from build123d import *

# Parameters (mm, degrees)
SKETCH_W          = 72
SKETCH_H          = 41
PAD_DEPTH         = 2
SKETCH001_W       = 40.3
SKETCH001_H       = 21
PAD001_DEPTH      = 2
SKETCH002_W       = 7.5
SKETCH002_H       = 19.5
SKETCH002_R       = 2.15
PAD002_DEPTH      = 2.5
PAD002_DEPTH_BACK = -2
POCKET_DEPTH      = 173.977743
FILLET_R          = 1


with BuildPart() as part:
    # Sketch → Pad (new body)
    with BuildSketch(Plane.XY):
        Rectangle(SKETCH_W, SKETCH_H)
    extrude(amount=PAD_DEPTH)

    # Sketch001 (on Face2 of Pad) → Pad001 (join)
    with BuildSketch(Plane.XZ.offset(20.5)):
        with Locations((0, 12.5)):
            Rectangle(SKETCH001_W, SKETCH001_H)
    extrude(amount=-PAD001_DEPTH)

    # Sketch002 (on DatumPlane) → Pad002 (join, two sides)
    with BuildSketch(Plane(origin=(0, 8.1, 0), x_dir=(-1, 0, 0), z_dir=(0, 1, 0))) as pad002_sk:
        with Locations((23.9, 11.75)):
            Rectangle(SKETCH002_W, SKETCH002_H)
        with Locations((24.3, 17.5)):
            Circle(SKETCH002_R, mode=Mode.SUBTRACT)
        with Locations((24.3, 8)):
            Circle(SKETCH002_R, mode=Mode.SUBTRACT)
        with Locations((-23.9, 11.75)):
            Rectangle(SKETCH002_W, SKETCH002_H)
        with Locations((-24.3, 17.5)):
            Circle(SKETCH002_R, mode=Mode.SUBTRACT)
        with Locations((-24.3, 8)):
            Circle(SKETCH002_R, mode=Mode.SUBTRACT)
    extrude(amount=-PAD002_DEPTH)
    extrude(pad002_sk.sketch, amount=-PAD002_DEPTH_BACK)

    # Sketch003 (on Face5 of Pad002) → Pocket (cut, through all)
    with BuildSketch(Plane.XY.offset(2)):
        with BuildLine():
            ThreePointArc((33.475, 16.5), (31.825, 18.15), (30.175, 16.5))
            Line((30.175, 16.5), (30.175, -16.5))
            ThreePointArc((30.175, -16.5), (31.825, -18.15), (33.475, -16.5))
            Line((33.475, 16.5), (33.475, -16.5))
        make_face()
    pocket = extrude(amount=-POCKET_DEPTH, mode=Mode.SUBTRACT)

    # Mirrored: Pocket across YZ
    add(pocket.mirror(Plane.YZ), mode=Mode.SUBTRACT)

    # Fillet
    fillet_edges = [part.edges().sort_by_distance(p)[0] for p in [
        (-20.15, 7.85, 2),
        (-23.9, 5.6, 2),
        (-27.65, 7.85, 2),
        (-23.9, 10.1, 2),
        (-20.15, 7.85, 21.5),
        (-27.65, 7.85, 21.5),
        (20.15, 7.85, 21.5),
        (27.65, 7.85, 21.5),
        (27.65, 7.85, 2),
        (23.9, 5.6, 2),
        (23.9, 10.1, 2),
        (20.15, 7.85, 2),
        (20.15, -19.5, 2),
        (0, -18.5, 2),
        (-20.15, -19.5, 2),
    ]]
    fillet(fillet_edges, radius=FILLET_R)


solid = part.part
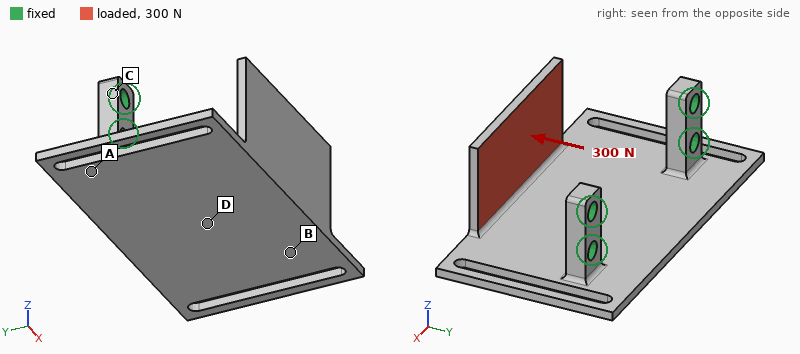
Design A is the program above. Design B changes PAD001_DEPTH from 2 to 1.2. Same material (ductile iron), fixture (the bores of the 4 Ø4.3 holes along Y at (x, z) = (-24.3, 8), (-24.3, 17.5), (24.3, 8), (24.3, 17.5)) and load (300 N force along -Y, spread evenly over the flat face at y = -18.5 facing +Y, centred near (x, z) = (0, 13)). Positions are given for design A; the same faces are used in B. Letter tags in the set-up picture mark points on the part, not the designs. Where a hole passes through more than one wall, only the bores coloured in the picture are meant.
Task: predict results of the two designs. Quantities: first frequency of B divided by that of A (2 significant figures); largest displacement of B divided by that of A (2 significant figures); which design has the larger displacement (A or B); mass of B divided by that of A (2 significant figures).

1.1
1.6
B
0.92
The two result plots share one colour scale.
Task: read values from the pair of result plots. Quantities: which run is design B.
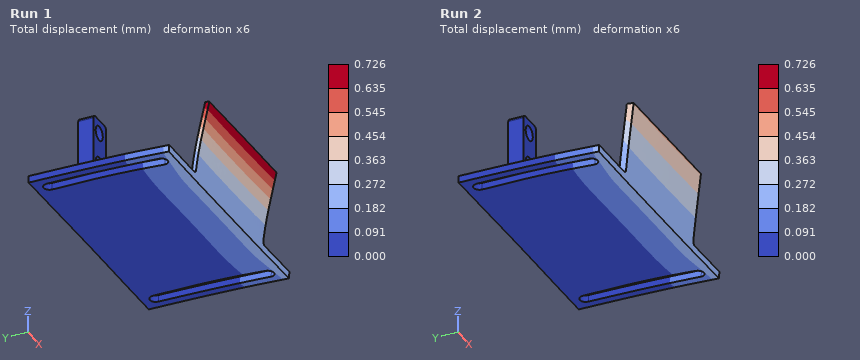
Run 1
